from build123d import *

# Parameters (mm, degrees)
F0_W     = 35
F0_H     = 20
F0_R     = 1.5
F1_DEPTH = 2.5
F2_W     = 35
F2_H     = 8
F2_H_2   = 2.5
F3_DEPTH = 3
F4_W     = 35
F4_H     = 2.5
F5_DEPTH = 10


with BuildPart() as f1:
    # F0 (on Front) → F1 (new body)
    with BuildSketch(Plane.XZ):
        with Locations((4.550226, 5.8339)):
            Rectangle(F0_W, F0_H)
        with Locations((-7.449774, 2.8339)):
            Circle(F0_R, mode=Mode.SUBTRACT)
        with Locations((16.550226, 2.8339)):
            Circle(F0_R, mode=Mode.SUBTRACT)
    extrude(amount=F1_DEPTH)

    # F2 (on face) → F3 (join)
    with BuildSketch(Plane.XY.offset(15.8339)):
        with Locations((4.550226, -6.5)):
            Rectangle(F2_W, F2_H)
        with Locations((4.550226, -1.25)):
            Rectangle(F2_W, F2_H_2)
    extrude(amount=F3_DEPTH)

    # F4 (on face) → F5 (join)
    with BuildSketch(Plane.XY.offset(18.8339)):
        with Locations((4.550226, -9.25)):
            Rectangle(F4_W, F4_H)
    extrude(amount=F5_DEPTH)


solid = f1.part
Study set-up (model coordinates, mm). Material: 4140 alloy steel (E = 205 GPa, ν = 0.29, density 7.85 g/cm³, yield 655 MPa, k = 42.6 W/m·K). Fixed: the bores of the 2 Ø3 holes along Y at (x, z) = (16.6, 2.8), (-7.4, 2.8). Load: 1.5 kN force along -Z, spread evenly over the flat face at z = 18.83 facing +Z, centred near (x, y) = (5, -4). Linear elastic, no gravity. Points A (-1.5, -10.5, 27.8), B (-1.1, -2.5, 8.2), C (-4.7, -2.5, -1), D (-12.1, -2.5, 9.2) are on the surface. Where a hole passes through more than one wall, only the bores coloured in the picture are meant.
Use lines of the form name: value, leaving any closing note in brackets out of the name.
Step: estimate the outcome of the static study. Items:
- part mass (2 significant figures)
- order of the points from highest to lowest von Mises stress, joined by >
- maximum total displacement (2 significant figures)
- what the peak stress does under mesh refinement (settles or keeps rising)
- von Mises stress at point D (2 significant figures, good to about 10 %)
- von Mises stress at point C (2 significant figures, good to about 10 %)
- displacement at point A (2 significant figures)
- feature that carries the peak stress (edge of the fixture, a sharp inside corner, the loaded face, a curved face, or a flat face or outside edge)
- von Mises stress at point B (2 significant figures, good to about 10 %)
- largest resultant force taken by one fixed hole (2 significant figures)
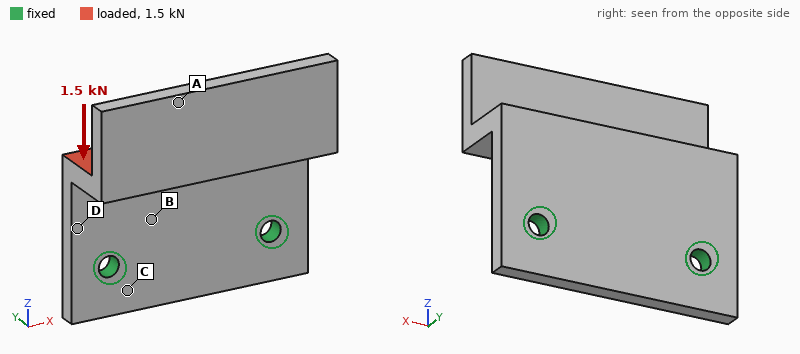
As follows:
part mass: 29 g
order of the points from highest to lowest von Mises stress, joined by >: D > B > C > A
maximum total displacement: 0.14 mm
what the peak stress does under mesh refinement: keeps rising
von Mises stress at point D: 140 MPa
von Mises stress at point C: 33 MPa
displacement at point A: 0.13 mm
feature that carries the peak stress: edge of the fixture
von Mises stress at point B: 110 MPa
largest resultant force taken by one fixed hole: 760 N
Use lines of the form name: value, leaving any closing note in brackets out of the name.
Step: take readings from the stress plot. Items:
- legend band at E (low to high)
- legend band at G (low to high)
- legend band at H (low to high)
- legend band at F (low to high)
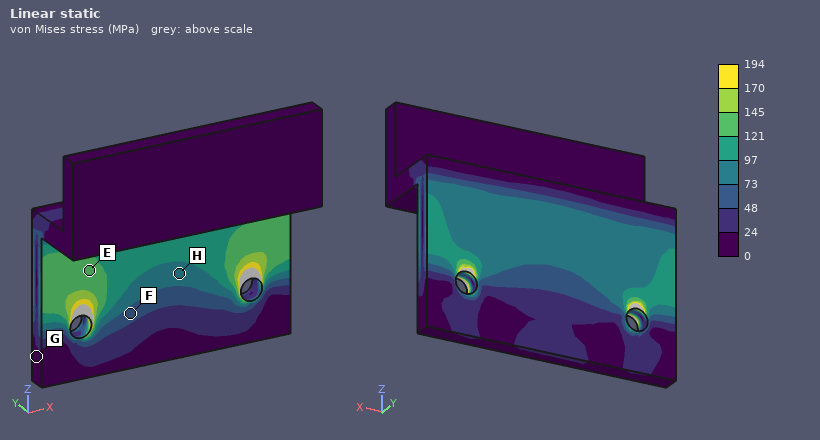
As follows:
legend band at E: 121 to 145 MPa
legend band at G: 0 to 24 MPa
legend band at H: 73 to 97 MPa
legend band at F: 48 to 73 MPa
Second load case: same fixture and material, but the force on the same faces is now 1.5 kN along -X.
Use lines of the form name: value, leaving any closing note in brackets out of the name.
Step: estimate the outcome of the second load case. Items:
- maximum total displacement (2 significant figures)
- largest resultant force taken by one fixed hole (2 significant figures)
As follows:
maximum total displacement: 26 µm
largest resultant force taken by one fixed hole: 1.2 kN
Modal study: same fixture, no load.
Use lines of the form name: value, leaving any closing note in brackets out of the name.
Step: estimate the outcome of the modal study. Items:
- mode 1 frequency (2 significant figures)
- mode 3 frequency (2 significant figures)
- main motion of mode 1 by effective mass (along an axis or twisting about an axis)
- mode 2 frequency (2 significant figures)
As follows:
mode 1 frequency: 2300 Hz
mode 3 frequency: 10 kHz
main motion of mode 1 by effective mass: along Y
mode 2 frequency: 5500 Hz
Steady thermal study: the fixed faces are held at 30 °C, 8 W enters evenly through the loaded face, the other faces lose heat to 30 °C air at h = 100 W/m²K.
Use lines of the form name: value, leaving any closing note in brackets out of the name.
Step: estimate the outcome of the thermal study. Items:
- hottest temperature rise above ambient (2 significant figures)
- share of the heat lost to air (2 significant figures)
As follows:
hottest temperature rise above ambient: 22 K
share of the heat lost to air: 48 %
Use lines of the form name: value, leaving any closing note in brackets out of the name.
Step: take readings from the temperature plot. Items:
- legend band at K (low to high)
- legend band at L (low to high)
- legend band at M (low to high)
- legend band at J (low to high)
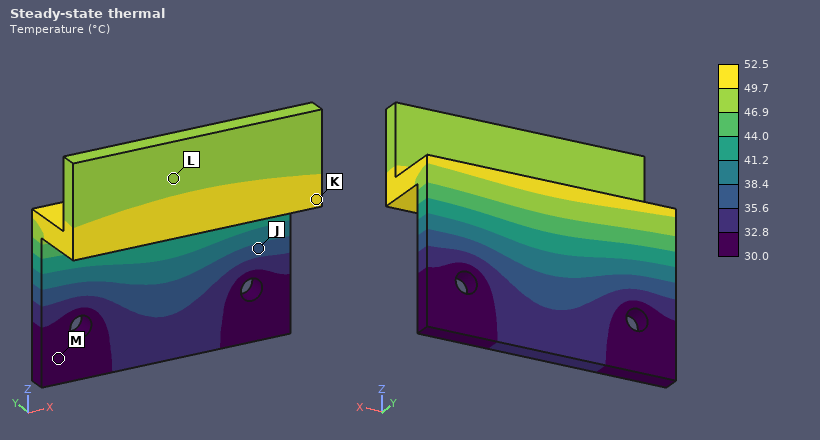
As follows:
legend band at K: 49.7 to 52.5 °C
legend band at L: 46.9 to 49.7 °C
legend band at M: 30.0 to 32.8 °C
legend band at J: 35.6 to 38.4 °C
